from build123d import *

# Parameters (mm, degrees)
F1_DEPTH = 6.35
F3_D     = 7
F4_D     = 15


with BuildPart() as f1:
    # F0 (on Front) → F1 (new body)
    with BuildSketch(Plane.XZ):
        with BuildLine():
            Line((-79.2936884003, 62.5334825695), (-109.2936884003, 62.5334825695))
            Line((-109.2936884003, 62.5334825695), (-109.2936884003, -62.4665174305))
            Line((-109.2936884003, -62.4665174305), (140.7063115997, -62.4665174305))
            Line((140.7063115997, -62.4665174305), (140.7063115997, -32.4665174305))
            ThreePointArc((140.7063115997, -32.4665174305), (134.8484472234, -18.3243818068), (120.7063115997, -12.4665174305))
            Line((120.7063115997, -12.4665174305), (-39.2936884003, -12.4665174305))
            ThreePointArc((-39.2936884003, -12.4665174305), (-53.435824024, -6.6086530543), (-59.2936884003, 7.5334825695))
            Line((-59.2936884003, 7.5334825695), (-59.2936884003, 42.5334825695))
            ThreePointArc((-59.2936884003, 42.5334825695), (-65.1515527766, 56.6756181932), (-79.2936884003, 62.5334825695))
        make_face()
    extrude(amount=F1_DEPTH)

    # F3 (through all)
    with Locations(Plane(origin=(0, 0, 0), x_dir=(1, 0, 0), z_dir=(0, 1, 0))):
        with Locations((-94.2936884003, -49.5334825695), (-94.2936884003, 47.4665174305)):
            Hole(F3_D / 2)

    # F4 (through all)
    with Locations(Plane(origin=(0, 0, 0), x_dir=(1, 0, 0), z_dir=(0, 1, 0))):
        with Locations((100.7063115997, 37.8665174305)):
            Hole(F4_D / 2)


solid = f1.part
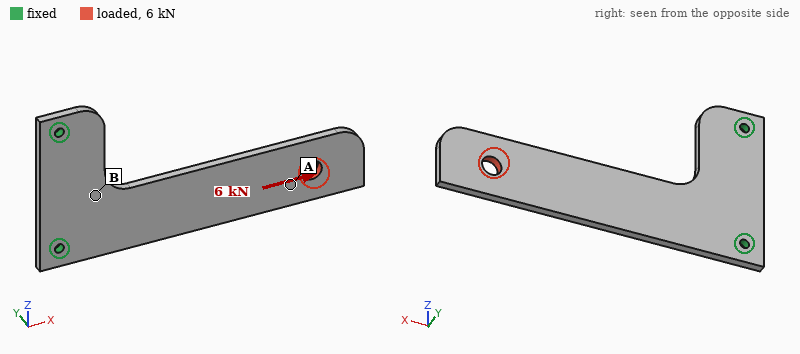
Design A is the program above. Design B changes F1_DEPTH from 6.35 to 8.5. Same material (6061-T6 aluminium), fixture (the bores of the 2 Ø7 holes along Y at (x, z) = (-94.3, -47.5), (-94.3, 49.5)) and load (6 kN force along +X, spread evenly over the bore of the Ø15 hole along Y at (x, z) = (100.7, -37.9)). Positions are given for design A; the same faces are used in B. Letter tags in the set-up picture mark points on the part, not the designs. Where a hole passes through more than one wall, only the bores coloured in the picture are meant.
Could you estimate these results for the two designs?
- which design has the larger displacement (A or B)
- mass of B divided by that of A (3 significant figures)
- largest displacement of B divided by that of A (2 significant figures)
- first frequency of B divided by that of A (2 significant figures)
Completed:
A
1.34
0.75
1.3
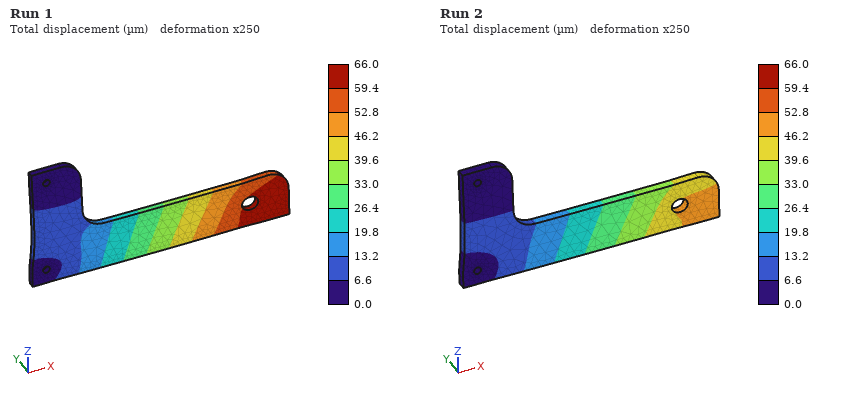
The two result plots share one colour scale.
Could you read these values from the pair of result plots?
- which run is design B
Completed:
Run 2
